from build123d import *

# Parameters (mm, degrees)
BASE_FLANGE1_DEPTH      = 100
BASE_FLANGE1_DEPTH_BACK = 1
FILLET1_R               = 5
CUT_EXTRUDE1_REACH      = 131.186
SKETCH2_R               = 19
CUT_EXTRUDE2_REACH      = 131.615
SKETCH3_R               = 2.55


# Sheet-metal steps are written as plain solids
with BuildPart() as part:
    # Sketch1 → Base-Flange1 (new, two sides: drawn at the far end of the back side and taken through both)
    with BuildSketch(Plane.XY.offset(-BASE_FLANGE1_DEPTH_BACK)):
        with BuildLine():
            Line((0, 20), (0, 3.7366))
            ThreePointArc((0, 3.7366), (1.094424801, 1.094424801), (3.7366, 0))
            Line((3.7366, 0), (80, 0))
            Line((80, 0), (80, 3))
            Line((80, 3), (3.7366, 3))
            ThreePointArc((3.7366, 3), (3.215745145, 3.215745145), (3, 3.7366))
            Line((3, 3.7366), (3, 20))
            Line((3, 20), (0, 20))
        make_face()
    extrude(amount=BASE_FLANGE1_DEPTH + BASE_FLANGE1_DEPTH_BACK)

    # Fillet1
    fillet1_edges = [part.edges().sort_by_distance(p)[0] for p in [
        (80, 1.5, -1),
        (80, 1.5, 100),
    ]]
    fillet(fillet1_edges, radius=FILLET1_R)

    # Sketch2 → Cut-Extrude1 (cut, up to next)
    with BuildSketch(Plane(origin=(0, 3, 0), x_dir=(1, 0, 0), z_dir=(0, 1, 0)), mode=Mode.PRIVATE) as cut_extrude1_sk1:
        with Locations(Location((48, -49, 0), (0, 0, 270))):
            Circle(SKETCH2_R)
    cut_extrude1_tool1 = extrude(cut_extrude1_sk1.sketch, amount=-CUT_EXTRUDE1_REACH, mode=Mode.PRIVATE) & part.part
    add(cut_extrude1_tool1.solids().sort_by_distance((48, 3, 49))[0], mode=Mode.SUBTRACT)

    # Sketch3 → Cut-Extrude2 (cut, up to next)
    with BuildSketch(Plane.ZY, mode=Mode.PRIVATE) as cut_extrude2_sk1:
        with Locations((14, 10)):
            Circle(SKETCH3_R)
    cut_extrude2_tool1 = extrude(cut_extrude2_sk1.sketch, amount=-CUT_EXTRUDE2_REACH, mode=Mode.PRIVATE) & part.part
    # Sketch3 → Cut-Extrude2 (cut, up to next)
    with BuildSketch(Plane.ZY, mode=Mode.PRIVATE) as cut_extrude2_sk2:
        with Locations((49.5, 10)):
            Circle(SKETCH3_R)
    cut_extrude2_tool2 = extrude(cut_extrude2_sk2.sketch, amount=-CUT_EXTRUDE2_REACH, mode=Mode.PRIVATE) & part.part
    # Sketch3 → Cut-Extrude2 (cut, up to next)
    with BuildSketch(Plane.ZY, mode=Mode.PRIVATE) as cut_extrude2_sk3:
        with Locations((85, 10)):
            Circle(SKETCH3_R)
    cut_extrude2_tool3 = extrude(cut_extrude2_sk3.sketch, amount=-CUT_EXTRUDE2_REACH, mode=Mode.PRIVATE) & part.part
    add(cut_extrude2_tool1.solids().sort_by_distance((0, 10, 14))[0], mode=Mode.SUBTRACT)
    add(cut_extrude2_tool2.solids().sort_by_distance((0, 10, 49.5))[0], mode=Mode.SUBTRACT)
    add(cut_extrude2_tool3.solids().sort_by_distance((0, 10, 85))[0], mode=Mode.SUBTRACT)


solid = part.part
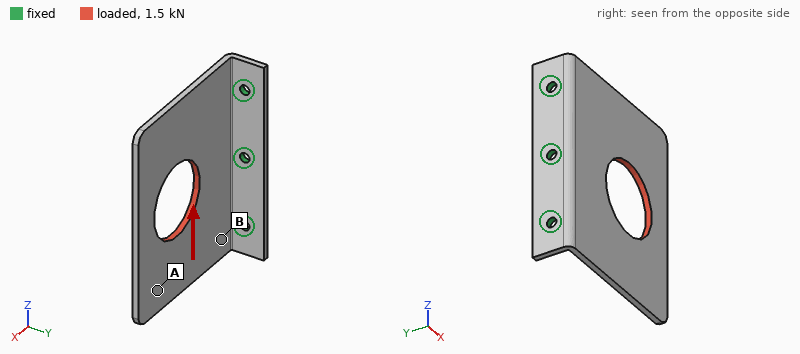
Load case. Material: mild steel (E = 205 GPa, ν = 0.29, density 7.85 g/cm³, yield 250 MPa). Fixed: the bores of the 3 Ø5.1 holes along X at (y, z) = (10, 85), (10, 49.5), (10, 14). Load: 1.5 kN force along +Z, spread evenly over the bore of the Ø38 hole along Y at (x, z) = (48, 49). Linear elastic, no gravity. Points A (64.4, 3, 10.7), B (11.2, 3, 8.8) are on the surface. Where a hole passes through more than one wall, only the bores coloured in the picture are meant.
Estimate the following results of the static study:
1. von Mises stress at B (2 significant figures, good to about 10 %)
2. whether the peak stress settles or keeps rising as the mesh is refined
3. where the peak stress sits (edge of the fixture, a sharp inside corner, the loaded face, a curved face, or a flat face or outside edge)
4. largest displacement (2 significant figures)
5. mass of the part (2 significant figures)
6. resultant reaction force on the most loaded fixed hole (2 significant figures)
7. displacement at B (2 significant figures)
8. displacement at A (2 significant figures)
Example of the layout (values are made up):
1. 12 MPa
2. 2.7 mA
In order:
1. 30 MPa
2. keeps rising
3. edge of the fixture
4. 76 µm
5. 200 g
6. 1.0 kN
7. 21 µm
8. 59 µm
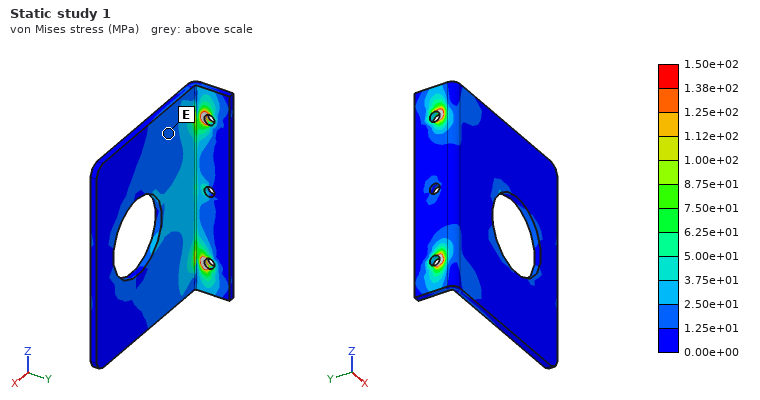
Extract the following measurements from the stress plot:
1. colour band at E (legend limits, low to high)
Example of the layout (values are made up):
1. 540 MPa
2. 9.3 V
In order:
1. 1.25e+01 to 2.50e+01 MPa
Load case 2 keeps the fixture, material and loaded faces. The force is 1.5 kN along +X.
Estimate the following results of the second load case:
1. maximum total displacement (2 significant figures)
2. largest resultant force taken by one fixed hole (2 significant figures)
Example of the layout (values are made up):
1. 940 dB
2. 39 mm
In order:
1. 97 µm
2. 520 N
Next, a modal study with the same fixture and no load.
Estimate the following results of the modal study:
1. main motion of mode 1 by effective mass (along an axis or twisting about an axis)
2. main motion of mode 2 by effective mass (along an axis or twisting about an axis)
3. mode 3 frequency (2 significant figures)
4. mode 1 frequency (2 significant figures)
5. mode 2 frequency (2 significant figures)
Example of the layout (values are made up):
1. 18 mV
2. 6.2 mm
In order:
1. along Y
2. twisting about X
3. 1900 Hz
4. 360 Hz
5. 700 Hz
